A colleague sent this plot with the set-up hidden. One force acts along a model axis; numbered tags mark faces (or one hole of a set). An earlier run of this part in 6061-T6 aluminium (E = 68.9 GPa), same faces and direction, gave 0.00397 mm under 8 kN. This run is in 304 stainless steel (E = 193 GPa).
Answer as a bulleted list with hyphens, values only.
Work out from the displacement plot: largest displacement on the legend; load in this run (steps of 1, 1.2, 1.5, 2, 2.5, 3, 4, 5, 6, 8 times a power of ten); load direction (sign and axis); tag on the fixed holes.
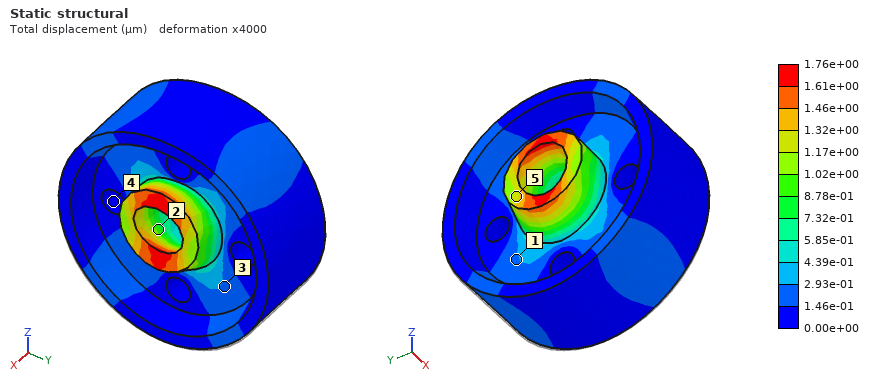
- 1.76e+00 µm
- 10 kN
- +Z
- 4
